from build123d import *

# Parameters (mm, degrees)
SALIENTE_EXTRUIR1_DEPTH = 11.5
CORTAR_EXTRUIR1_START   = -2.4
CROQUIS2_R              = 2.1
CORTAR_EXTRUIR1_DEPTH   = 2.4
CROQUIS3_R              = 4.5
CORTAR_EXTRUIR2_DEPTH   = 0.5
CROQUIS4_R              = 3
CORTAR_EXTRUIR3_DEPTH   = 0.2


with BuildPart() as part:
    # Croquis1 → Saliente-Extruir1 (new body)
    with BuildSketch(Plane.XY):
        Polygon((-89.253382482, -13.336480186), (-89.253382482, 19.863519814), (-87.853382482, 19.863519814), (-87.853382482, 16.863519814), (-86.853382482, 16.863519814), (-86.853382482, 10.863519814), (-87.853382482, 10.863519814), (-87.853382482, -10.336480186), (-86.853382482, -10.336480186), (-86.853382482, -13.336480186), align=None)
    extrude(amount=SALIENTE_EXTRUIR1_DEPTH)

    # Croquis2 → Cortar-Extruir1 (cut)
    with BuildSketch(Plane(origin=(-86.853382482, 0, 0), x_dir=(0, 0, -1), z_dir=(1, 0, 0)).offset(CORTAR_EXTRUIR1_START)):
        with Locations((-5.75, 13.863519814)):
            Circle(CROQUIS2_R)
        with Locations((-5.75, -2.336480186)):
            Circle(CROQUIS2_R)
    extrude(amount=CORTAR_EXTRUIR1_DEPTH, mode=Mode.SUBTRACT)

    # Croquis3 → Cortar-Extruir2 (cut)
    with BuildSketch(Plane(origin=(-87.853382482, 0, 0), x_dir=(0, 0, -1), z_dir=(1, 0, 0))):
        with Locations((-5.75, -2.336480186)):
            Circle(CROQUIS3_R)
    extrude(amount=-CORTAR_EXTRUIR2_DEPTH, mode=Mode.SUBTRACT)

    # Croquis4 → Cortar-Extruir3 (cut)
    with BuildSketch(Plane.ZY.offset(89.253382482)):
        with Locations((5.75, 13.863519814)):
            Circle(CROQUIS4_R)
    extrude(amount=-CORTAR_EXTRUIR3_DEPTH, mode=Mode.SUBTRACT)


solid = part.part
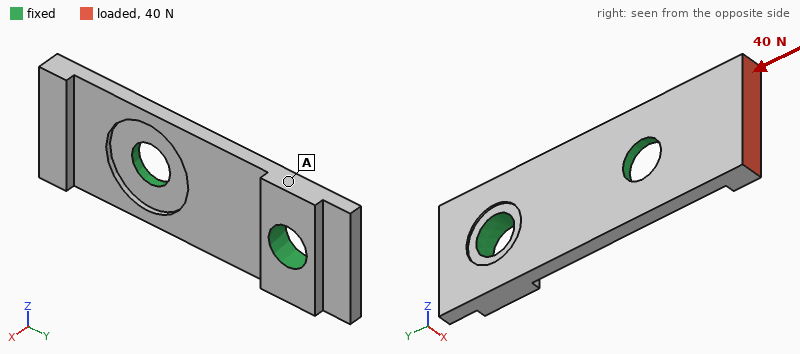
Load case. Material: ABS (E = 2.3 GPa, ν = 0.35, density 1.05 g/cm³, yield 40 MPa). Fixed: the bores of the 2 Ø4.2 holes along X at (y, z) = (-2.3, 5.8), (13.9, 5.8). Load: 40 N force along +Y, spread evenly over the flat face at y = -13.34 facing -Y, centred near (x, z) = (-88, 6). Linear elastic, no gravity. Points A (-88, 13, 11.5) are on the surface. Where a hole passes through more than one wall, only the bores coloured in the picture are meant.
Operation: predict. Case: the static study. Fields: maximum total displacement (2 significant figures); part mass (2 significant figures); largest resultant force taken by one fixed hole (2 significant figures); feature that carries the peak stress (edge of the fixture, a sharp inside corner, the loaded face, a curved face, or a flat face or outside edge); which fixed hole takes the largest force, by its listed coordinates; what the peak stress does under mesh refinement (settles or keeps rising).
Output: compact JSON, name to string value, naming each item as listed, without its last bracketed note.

{"maximum total displacement": "0.31 mm", "part mass": "0.59 g", "largest resultant force taken by one fixed hole": "34 N", "feature that carries the peak stress": "edge of the fixture", "which fixed hole takes the largest force, by its listed coordinates": "(-2.3, 5.8)", "what the peak stress does under mesh refinement": "keeps rising"}
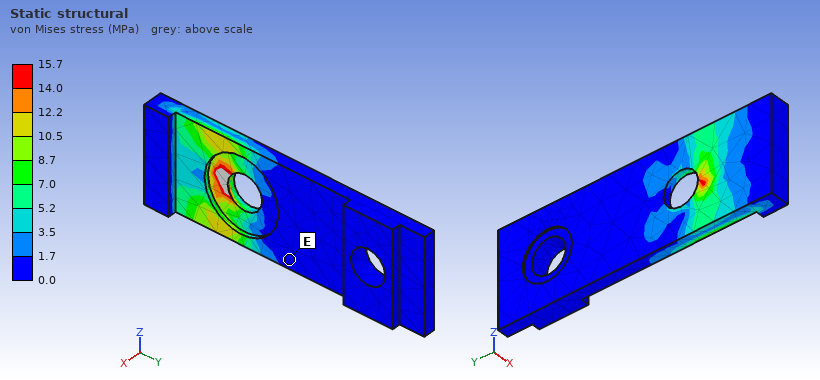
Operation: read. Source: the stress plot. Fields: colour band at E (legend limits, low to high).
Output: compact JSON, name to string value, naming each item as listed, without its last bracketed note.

{"colour band at E": "0.0 to 1.7 MPa"}
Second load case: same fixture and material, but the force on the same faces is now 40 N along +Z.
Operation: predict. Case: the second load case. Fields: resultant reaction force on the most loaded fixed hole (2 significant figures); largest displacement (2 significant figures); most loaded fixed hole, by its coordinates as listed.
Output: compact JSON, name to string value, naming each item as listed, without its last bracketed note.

{"resultant reaction force on the most loaded fixed hole": "52 N", "largest displacement": "0.19 mm", "most loaded fixed hole, by its coordinates as listed": "(-2.3, 5.8)"}
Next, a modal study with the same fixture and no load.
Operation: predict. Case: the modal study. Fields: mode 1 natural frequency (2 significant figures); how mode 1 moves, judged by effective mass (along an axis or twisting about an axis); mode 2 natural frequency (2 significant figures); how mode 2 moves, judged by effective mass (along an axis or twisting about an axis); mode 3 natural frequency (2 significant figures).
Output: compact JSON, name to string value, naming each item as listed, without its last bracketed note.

{"mode 1 natural frequency": "2000 Hz", "how mode 1 moves, judged by effective mass": "along X", "mode 2 natural frequency": "4200 Hz", "how mode 2 moves, judged by effective mass": "twisting about Y", "mode 3 natural frequency": "9100 Hz"}
